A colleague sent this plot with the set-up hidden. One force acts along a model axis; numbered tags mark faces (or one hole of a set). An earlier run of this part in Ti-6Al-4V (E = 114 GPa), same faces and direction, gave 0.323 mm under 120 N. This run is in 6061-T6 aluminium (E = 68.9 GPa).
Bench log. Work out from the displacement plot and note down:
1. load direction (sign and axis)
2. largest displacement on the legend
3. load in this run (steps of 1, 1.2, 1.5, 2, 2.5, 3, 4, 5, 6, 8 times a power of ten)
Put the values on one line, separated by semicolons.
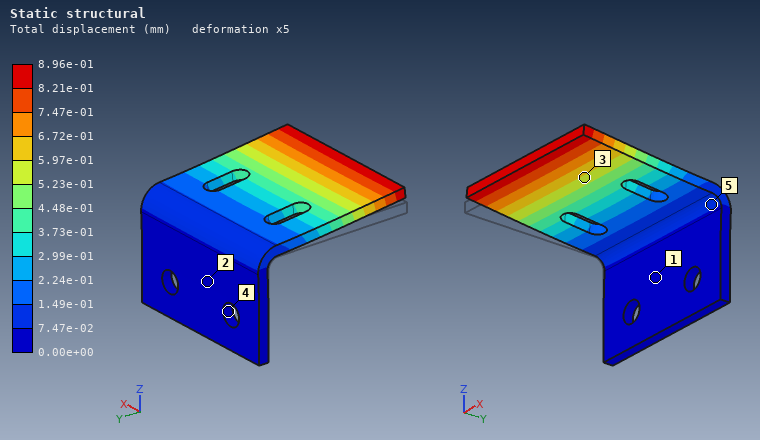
+Z; 8.96e-01 mm; 200 N
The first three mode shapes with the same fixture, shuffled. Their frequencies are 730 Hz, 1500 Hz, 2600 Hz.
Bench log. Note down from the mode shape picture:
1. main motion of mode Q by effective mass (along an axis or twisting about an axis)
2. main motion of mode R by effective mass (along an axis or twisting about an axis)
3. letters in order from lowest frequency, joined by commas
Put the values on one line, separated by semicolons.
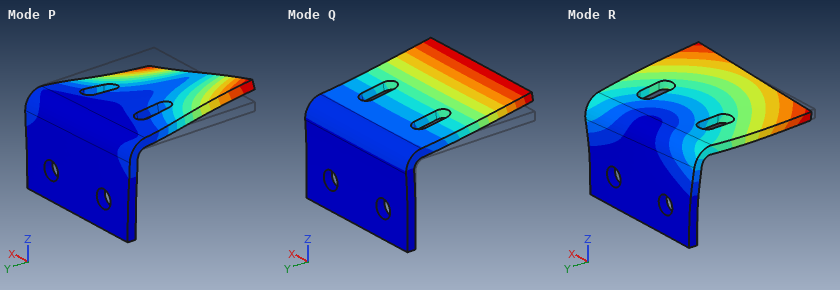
along Z; along X; Q, R, P
